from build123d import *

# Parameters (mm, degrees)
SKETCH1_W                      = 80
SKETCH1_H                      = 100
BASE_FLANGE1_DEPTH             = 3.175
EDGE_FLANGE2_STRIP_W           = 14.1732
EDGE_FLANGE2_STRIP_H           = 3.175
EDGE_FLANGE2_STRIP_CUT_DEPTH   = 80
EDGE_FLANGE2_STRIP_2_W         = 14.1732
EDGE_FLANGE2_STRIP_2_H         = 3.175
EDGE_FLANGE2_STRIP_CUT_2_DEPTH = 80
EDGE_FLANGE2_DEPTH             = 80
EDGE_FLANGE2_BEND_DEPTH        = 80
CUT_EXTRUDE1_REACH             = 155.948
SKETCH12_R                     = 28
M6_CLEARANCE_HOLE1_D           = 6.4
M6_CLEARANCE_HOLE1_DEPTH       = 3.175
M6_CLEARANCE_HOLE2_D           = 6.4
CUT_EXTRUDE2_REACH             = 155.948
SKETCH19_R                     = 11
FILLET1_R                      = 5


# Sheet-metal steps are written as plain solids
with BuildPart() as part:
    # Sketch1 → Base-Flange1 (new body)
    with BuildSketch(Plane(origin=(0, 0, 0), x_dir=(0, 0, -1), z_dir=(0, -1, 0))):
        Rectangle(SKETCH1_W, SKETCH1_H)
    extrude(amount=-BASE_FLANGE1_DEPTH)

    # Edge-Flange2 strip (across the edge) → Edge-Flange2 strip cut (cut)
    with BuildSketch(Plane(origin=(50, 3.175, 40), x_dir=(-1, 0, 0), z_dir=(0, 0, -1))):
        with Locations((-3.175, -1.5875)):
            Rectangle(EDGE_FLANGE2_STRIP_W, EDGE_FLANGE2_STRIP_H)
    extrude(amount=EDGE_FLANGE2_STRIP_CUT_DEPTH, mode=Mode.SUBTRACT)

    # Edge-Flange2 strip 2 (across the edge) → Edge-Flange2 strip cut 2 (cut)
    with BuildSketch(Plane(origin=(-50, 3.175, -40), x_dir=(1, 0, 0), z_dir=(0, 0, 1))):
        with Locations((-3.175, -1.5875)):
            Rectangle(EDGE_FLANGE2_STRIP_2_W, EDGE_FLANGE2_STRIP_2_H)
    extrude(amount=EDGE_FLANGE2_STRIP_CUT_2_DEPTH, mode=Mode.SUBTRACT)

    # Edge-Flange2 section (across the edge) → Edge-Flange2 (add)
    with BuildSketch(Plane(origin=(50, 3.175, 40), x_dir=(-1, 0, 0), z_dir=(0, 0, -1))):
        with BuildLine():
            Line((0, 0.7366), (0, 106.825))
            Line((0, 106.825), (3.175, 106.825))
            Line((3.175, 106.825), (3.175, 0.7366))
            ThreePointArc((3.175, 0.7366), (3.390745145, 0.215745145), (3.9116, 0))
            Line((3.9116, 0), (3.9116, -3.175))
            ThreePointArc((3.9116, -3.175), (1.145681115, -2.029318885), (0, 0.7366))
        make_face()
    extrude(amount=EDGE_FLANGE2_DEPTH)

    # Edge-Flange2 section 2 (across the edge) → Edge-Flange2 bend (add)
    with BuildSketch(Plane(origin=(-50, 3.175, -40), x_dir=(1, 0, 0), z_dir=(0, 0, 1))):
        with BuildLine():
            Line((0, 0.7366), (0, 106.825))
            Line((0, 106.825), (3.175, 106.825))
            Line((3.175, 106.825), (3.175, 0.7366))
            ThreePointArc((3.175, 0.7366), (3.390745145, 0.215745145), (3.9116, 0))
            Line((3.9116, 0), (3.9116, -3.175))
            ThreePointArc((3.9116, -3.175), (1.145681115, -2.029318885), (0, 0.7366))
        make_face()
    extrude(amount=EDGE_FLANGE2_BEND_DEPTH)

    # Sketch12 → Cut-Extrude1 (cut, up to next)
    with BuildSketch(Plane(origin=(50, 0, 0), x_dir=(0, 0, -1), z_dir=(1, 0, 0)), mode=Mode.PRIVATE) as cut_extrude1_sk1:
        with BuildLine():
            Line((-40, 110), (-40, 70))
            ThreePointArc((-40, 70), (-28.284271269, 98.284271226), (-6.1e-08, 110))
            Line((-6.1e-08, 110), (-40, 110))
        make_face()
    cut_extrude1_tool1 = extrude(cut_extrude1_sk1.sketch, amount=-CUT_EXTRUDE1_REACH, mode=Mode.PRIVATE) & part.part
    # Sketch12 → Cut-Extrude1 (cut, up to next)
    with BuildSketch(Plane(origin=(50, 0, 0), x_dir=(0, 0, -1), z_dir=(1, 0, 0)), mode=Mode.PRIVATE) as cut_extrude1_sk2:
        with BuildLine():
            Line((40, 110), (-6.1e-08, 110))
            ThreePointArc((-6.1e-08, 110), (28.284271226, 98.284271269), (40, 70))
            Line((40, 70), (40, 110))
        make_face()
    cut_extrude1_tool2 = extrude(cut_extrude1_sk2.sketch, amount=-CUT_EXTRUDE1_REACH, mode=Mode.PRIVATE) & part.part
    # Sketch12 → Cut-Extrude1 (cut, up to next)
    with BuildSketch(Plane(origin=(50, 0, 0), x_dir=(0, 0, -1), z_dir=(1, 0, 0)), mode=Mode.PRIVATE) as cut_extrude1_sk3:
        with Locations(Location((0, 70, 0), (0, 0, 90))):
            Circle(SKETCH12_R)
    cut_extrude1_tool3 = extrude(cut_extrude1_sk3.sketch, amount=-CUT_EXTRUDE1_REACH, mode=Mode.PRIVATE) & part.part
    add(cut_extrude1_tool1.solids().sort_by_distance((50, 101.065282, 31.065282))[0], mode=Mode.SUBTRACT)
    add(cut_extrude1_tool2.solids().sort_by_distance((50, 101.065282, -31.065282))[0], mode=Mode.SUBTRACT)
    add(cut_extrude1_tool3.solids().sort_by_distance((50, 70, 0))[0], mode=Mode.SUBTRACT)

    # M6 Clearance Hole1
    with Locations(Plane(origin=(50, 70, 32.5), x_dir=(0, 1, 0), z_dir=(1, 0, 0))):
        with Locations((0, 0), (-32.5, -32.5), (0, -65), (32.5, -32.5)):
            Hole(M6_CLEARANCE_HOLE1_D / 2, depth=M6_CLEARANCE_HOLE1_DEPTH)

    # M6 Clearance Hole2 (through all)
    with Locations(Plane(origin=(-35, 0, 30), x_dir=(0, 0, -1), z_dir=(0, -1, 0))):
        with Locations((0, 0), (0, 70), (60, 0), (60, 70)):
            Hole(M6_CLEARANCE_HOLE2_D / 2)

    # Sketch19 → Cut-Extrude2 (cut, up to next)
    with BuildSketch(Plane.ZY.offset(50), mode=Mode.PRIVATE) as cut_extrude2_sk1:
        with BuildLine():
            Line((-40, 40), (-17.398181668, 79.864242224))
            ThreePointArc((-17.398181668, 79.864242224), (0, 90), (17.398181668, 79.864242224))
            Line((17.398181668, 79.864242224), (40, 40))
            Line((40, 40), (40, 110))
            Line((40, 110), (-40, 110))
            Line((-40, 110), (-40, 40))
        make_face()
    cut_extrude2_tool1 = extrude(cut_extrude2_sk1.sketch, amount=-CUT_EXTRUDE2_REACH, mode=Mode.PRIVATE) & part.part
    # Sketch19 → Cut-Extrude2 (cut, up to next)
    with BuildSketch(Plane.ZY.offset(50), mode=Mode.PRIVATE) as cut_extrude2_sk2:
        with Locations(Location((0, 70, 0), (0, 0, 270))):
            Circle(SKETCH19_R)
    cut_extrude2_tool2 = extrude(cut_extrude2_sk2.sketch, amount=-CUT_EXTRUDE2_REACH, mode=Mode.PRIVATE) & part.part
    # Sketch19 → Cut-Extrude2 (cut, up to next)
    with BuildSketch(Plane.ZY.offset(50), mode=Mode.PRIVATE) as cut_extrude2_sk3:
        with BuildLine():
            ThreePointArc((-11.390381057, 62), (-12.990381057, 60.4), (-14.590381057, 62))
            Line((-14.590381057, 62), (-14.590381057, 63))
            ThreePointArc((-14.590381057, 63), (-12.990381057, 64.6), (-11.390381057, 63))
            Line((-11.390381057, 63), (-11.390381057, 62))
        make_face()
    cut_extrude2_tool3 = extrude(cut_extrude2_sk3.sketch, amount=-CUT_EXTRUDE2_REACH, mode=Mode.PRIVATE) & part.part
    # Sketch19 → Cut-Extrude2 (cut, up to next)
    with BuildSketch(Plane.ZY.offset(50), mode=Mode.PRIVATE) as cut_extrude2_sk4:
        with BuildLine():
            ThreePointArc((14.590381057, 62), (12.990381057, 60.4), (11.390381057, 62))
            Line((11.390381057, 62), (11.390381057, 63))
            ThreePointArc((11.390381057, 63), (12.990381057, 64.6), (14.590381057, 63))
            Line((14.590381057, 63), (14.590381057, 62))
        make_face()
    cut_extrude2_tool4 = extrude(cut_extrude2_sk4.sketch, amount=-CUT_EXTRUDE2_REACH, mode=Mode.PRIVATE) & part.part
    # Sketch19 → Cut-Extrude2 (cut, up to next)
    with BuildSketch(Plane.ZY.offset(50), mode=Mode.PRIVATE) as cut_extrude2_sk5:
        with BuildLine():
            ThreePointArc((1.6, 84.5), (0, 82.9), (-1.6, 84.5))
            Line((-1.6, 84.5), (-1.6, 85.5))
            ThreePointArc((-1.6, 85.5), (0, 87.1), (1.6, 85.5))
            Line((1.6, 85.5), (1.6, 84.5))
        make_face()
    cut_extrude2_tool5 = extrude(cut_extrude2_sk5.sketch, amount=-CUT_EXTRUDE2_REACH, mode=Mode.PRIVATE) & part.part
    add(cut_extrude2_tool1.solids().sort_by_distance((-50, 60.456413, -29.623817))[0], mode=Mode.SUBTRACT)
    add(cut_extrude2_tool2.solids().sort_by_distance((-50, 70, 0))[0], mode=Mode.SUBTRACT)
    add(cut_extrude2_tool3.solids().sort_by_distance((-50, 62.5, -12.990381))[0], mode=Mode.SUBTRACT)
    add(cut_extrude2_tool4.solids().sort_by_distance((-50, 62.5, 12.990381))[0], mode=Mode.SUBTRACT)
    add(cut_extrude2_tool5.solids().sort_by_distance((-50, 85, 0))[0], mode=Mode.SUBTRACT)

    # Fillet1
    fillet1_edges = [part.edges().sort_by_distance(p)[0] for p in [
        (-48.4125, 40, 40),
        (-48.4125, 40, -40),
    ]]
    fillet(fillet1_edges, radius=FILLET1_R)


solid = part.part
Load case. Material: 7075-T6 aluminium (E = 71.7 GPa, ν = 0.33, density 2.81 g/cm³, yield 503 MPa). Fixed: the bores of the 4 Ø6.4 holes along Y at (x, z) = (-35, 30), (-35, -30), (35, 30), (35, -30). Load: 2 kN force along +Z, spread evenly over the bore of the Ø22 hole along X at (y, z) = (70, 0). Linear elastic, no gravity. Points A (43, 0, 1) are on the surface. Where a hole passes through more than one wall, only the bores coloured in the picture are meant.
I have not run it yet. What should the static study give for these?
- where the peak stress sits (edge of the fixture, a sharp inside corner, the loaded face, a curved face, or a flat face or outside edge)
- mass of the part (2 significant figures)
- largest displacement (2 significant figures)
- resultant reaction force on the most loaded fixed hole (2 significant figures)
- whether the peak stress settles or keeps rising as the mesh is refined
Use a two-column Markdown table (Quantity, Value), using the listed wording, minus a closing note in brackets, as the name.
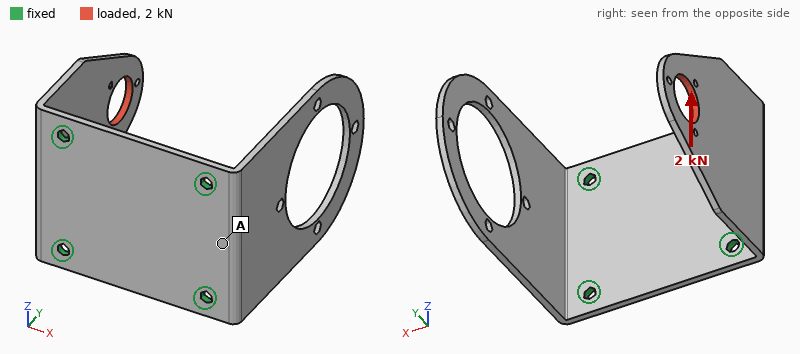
| Quantity | Value |
|---|---|
| where the peak stress sits | edge of the fixture |
| mass of the part | 160 g |
| largest displacement | 0.67 mm |
| resultant reaction force on the most loaded fixed hole | 2.5 kN |
| whether the peak stress settles or keeps rising as the mesh is refined | keeps rising |
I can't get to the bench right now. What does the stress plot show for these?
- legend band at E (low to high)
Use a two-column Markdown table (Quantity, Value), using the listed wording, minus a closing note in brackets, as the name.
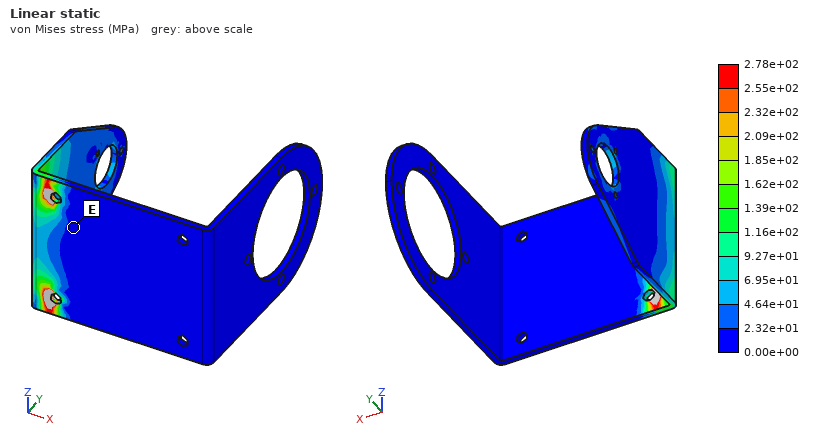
| Quantity | Value |
|---|---|
| legend band at E | 0.00e+00 to 2.32e+01 MPa |
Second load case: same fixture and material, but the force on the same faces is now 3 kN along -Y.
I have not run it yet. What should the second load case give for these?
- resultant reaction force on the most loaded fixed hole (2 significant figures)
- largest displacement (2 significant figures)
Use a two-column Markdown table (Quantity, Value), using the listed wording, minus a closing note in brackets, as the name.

| Quantity | Value |
|---|---|
| resultant reaction force on the most loaded fixed hole | 1.6 kN |
| largest displacement | 1.5 mm |
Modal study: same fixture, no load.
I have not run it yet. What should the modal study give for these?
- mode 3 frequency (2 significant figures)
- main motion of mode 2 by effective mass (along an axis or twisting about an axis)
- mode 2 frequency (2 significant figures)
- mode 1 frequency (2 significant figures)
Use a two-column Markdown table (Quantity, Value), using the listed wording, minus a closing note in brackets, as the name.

| Quantity | Value |
|---|---|
| mode 3 frequency | 720 Hz |
| main motion of mode 2 by effective mass | along X |
| mode 2 frequency | 410 Hz |
| mode 1 frequency | 270 Hz |
